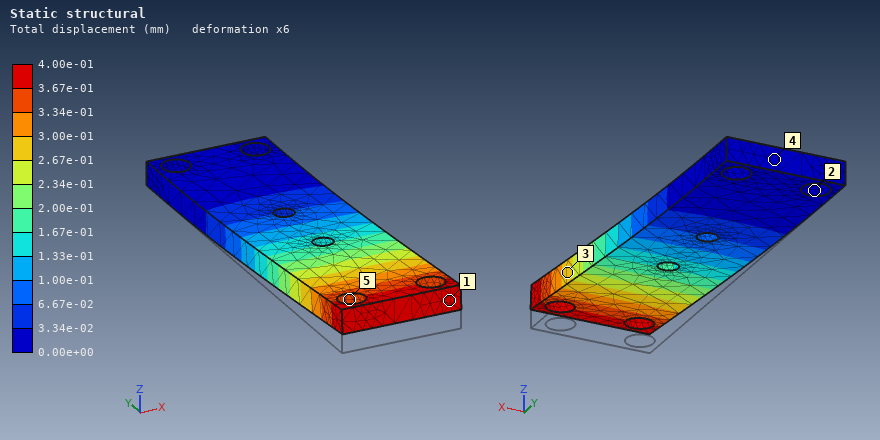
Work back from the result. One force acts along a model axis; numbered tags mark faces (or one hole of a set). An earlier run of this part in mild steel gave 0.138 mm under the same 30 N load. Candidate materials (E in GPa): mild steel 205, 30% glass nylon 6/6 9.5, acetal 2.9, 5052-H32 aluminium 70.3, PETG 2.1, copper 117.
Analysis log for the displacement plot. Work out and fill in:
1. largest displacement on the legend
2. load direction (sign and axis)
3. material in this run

4.00e-01 mm
+Z
5052-H32 aluminium
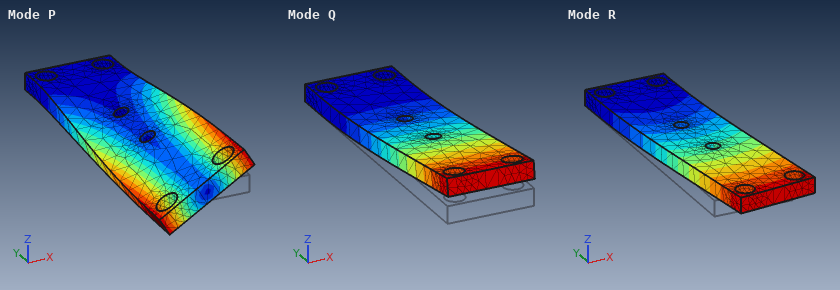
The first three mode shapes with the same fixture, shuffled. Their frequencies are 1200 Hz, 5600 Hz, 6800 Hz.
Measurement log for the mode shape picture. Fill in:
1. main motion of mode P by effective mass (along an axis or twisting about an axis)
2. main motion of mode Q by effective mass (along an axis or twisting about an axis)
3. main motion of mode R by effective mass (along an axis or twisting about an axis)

twisting about Y
along Z
along X
